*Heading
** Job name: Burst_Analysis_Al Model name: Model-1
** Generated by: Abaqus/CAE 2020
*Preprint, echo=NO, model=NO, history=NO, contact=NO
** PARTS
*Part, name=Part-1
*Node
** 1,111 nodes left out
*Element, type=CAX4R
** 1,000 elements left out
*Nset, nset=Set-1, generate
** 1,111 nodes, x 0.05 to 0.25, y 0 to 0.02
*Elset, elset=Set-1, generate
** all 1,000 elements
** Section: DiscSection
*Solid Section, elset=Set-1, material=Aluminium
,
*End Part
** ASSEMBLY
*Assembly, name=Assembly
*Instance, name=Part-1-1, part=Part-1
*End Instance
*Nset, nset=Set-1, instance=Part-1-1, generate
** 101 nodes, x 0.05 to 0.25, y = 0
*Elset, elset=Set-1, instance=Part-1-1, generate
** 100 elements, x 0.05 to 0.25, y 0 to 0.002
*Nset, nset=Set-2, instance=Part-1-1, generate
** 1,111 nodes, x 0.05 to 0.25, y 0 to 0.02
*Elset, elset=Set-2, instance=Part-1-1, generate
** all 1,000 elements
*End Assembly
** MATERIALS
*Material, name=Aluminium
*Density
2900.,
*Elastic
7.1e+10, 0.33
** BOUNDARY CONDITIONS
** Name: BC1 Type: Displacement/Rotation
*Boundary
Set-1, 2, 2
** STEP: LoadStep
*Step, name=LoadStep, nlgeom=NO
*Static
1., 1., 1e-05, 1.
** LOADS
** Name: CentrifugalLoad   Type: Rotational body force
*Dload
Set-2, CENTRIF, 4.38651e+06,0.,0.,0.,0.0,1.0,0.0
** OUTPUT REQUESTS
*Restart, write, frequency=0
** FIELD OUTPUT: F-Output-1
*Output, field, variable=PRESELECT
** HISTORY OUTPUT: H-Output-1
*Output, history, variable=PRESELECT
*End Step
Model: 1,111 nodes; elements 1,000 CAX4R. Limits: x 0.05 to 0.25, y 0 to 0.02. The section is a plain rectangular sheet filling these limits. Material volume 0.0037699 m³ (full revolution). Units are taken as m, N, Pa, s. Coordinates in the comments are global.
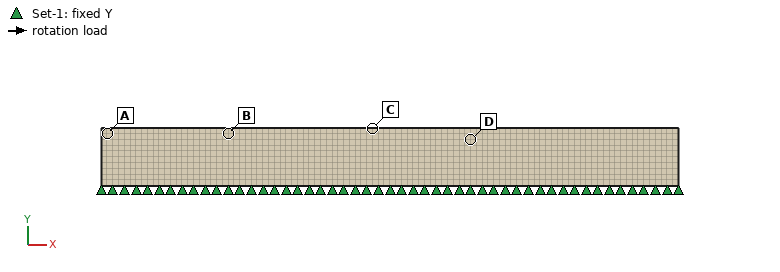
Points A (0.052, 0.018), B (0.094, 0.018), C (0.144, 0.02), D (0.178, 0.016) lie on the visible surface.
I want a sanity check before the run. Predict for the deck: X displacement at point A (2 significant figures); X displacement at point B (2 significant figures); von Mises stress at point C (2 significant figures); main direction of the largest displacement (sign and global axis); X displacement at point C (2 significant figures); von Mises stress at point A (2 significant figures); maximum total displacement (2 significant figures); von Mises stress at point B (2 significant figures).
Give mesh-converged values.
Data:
4.6e-04 m
4.5e-04 m
2.8e+08 Pa
+X
5.1e-04 m
6.3e+08 Pa
5.7e-04 m
3.5e+08 Pa
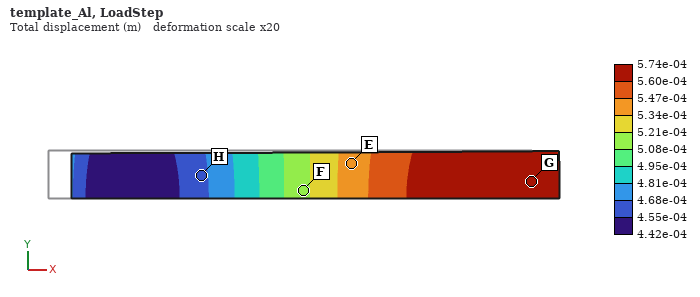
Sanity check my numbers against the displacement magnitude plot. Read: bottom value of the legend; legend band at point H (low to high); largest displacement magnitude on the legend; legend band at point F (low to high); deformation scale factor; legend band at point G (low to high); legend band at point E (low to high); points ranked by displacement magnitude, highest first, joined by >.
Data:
4.42e-04 m
4.55e-04 to 4.68e-04 m
5.74e-04 m
5.08e-04 to 5.21e-04 m
20
5.60e-04 to 5.74e-04 m
5.34e-04 to 5.47e-04 m
G > E > F > H
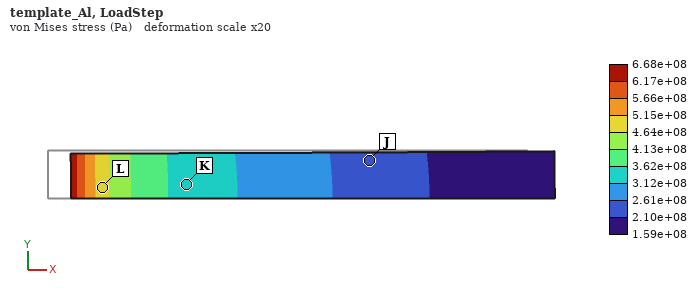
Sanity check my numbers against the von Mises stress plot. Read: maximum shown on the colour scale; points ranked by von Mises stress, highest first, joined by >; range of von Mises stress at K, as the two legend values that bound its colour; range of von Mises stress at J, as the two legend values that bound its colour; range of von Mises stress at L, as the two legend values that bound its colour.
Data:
6.68e+08 Pa
L > K > J
3.12e+08 to 3.62e+08 Pa
2.10e+08 to 2.61e+08 Pa
4.64e+08 to 5.15e+08 Pa
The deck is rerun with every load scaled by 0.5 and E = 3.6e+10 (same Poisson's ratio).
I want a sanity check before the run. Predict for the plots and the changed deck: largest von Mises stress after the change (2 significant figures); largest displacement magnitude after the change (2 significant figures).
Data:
3.3e+08 Pa
5.7e-04 m
